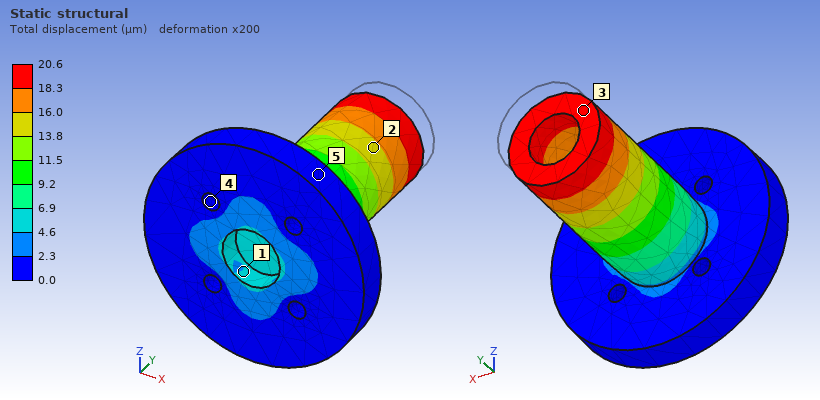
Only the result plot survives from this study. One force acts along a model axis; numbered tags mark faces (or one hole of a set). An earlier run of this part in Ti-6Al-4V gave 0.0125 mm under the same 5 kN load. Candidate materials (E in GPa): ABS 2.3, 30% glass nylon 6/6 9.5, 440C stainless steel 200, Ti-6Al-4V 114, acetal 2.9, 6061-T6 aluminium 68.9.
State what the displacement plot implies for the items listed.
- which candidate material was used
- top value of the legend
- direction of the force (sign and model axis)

6061-T6 aluminium
20.6 µm
-Y
